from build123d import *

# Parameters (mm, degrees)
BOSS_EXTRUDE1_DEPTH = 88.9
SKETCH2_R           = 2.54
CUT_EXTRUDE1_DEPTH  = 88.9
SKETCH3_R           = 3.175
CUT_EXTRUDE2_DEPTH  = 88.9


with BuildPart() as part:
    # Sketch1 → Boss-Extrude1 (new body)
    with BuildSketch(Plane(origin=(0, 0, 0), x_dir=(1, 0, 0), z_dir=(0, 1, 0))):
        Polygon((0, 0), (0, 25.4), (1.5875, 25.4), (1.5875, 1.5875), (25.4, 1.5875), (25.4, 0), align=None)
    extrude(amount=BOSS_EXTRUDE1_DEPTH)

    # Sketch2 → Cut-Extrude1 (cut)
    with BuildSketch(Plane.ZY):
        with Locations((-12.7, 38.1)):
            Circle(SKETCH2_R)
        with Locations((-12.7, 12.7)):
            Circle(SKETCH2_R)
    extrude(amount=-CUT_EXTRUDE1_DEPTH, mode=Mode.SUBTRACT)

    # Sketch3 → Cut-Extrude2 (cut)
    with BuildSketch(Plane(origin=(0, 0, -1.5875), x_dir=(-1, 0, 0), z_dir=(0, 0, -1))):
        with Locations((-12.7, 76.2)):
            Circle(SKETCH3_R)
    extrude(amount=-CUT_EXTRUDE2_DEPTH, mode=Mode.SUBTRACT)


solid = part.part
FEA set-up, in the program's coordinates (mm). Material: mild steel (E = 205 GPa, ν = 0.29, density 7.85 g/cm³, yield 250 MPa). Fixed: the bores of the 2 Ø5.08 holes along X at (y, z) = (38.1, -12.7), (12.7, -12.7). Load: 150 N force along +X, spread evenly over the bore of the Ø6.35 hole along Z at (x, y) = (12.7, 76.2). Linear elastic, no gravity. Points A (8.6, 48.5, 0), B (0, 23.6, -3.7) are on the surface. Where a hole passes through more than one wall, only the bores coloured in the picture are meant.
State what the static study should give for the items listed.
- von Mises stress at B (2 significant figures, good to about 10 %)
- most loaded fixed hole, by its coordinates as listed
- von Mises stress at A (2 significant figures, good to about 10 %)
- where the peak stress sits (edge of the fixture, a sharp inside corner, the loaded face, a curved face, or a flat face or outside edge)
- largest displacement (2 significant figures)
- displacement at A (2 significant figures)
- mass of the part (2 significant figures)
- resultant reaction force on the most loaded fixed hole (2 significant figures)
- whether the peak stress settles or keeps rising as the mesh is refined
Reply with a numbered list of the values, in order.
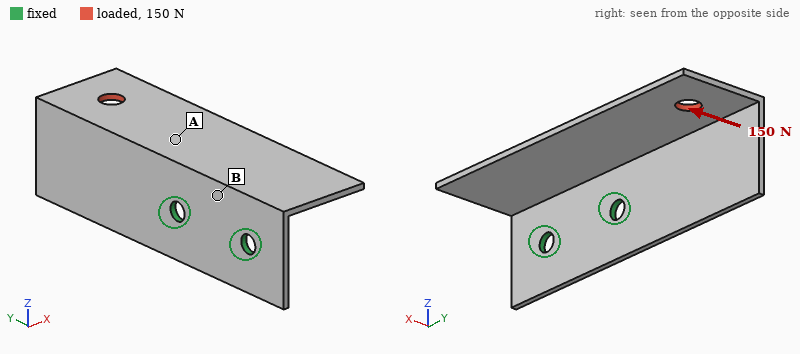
1. 68 MPa
2. (38.1, -12.7)
3. 29 MPa
4. edge of the fixture
5. 0.27 mm
6. 0.10 mm
7. 54 g
8. 320 N
9. keeps rising
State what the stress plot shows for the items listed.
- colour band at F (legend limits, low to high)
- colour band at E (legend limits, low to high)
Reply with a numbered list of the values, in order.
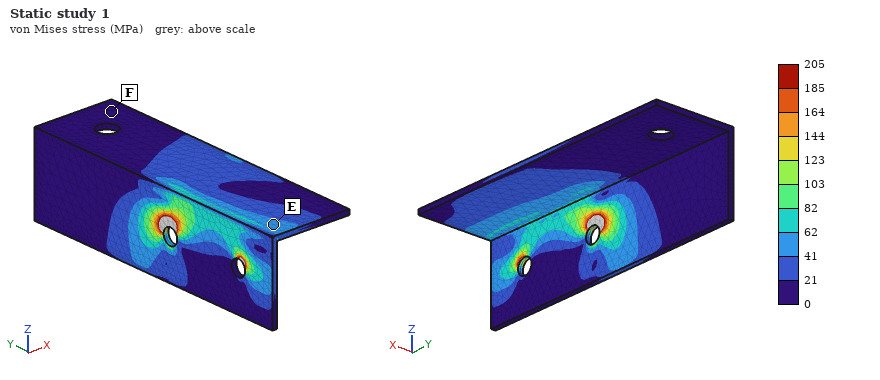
1. 0 to 21 MPa
2. 41 to 62 MPa
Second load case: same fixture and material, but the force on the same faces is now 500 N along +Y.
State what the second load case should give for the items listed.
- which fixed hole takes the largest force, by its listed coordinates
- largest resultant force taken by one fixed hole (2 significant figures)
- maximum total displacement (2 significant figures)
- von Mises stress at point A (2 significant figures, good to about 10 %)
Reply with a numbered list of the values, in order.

1. (38.1, -12.7)
2. 390 N
3. 0.18 mm
4. 23 MPa
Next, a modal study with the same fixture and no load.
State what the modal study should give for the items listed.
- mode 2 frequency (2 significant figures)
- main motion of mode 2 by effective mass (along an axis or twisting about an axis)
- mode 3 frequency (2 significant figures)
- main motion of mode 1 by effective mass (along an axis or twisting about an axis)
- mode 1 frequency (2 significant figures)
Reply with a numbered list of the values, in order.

1. 1100 Hz
2. along X
3. 1600 Hz
4. along Z
5. 940 Hz
